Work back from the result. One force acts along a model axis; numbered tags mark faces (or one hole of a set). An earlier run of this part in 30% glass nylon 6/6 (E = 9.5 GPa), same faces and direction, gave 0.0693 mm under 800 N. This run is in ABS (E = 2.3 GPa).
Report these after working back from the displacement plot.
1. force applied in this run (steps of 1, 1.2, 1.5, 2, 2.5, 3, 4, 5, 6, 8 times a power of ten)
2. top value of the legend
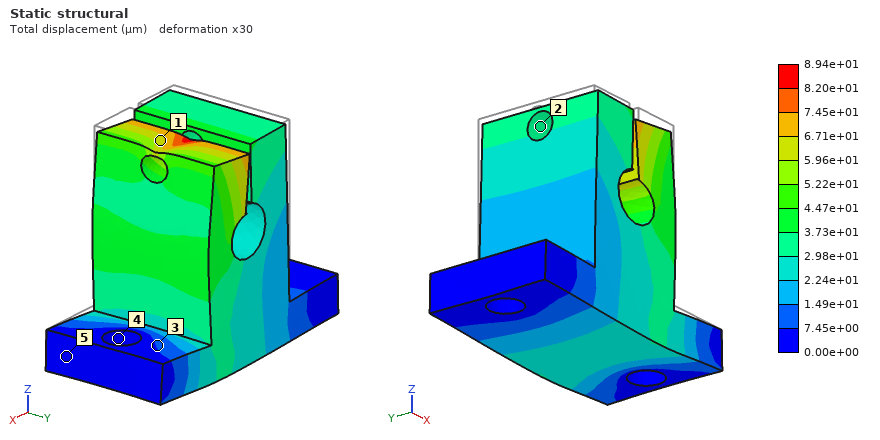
250 N
8.94e+01 µm
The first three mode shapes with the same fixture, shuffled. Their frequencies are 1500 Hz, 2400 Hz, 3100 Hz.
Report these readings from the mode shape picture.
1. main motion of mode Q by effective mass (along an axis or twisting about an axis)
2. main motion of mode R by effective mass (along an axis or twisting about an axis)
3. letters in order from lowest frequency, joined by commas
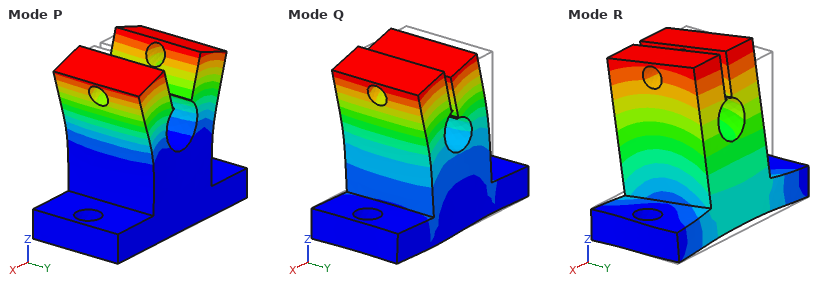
along X
along Y
R, Q, P
